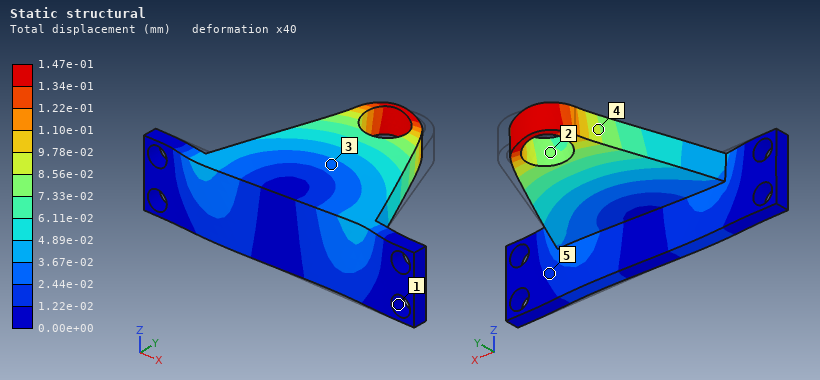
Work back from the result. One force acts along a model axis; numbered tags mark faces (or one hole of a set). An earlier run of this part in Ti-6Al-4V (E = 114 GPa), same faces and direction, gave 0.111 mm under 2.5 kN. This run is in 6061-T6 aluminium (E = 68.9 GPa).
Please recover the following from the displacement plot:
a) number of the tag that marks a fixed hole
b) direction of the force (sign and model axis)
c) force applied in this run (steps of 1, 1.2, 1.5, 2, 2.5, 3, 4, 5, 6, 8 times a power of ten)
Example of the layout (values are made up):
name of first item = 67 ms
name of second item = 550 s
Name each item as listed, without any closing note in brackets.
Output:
number of the tag that marks a fixed hole = 1
direction of the force = -X
force applied in this run = 2 kN
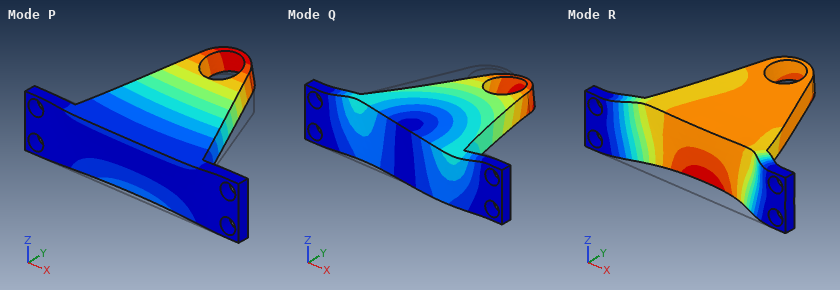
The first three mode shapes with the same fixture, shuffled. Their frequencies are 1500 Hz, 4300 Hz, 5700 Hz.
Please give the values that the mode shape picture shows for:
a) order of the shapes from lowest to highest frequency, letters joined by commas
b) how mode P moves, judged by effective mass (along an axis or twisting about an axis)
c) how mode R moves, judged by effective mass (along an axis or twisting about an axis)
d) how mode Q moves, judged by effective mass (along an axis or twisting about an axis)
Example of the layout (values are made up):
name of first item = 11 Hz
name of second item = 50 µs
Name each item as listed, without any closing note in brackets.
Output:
order of the shapes from lowest to highest frequency, letters joined by commas = P, R, Q
how mode P moves, judged by effective mass = along Z
how mode R moves, judged by effective mass = along Y
how mode Q moves, judged by effective mass = along X
